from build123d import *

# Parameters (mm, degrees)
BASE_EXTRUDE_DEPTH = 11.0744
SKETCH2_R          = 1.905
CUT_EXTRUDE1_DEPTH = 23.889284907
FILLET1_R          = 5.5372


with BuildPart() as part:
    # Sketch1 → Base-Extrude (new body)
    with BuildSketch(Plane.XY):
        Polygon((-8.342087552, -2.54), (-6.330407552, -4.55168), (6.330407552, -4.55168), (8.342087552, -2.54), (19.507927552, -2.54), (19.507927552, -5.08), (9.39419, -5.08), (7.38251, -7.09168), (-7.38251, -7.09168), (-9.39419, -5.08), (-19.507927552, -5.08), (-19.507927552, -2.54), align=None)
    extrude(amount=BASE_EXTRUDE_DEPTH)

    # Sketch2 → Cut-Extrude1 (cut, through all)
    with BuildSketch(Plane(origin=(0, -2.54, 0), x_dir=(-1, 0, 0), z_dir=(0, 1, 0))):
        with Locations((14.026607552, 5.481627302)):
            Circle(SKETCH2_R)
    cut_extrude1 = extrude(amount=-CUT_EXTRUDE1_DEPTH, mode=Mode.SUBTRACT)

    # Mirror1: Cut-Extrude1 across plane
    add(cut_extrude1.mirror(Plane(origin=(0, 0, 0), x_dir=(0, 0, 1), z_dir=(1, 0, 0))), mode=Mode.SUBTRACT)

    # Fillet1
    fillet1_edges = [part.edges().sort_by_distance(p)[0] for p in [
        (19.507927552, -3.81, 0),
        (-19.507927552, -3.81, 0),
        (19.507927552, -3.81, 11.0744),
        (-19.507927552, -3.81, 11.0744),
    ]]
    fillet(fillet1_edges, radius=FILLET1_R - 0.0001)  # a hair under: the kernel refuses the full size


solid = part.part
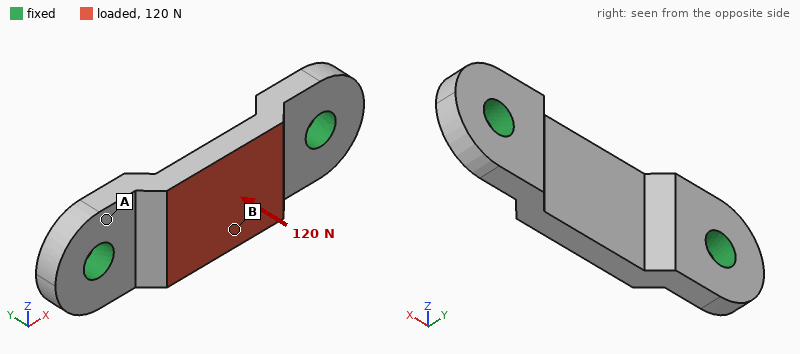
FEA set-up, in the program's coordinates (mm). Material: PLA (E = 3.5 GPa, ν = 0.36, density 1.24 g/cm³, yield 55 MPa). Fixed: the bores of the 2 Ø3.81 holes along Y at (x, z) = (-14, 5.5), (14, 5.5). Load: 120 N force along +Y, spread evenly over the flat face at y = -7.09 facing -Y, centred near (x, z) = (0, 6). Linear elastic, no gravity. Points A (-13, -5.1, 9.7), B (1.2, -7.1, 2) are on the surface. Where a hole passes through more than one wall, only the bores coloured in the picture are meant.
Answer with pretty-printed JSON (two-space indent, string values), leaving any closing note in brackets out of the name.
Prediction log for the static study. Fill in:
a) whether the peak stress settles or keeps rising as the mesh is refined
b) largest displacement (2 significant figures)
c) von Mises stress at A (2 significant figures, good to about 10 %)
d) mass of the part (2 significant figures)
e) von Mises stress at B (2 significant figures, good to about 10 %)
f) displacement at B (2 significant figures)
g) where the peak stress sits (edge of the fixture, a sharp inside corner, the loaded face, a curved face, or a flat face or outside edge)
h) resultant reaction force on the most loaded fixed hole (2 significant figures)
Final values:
{
  "whether the peak stress settles or keeps rising as the mesh is refined": "keeps rising",
  "largest displacement": "0.10 mm",
  "von Mises stress at A": "4.2 MPa",
  "mass of the part": "1.3 g",
  "von Mises stress at B": "13 MPa",
  "displacement at B": "0.091 mm",
  "where the peak stress sits": "edge of the fixture",
  "resultant reaction force on the most loaded fixed hole": "120 N"
}
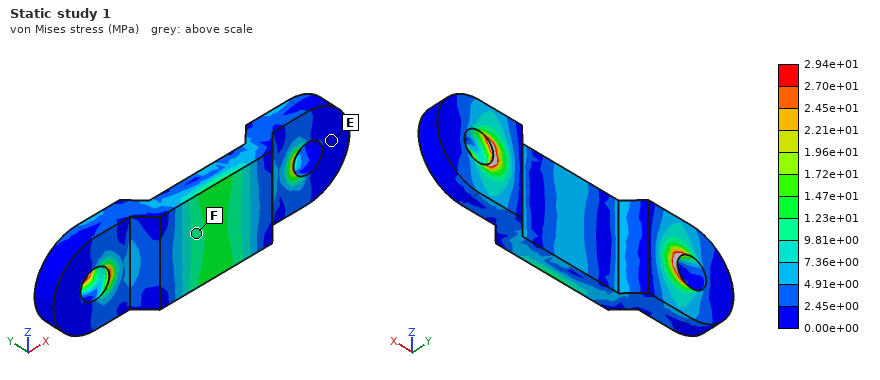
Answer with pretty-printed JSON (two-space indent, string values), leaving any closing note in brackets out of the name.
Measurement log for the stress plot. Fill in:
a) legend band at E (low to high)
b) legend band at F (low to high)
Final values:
{
  "legend band at E": "0.00e+00 to 2.45e+00 MPa",
  "legend band at F": "9.81e+00 to 1.23e+01 MPa"
}
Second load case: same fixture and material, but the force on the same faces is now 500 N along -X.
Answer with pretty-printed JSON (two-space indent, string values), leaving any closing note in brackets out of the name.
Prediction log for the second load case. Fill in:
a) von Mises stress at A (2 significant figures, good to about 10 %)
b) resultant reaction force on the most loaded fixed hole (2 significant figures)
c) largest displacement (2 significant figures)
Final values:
{
  "von Mises stress at A": "5.2 MPa",
  "resultant reaction force on the most loaded fixed hole": "260 N",
  "largest displacement": "45 µm"
}
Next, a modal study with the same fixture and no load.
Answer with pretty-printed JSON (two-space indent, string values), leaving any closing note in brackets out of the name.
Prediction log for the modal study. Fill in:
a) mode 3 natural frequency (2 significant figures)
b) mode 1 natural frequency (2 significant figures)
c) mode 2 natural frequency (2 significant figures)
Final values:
{
  "mode 3 natural frequency": "14 kHz",
  "mode 1 natural frequency": "8100 Hz",
  "mode 2 natural frequency": "8200 Hz"
}
